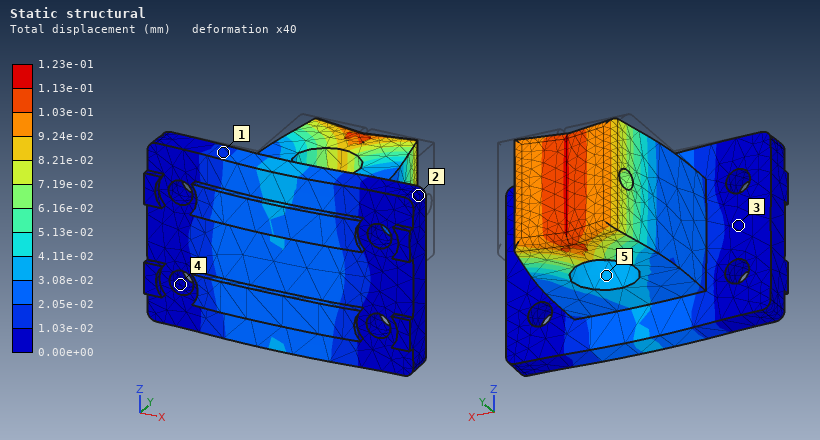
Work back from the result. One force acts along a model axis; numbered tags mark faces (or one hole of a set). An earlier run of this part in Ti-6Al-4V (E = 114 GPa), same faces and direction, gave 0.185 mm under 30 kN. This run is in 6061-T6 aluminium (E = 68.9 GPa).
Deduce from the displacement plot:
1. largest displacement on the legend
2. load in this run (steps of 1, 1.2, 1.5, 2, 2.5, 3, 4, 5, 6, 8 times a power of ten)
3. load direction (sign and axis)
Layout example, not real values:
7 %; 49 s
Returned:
1.23e-01 mm; 12 kN; -Y
